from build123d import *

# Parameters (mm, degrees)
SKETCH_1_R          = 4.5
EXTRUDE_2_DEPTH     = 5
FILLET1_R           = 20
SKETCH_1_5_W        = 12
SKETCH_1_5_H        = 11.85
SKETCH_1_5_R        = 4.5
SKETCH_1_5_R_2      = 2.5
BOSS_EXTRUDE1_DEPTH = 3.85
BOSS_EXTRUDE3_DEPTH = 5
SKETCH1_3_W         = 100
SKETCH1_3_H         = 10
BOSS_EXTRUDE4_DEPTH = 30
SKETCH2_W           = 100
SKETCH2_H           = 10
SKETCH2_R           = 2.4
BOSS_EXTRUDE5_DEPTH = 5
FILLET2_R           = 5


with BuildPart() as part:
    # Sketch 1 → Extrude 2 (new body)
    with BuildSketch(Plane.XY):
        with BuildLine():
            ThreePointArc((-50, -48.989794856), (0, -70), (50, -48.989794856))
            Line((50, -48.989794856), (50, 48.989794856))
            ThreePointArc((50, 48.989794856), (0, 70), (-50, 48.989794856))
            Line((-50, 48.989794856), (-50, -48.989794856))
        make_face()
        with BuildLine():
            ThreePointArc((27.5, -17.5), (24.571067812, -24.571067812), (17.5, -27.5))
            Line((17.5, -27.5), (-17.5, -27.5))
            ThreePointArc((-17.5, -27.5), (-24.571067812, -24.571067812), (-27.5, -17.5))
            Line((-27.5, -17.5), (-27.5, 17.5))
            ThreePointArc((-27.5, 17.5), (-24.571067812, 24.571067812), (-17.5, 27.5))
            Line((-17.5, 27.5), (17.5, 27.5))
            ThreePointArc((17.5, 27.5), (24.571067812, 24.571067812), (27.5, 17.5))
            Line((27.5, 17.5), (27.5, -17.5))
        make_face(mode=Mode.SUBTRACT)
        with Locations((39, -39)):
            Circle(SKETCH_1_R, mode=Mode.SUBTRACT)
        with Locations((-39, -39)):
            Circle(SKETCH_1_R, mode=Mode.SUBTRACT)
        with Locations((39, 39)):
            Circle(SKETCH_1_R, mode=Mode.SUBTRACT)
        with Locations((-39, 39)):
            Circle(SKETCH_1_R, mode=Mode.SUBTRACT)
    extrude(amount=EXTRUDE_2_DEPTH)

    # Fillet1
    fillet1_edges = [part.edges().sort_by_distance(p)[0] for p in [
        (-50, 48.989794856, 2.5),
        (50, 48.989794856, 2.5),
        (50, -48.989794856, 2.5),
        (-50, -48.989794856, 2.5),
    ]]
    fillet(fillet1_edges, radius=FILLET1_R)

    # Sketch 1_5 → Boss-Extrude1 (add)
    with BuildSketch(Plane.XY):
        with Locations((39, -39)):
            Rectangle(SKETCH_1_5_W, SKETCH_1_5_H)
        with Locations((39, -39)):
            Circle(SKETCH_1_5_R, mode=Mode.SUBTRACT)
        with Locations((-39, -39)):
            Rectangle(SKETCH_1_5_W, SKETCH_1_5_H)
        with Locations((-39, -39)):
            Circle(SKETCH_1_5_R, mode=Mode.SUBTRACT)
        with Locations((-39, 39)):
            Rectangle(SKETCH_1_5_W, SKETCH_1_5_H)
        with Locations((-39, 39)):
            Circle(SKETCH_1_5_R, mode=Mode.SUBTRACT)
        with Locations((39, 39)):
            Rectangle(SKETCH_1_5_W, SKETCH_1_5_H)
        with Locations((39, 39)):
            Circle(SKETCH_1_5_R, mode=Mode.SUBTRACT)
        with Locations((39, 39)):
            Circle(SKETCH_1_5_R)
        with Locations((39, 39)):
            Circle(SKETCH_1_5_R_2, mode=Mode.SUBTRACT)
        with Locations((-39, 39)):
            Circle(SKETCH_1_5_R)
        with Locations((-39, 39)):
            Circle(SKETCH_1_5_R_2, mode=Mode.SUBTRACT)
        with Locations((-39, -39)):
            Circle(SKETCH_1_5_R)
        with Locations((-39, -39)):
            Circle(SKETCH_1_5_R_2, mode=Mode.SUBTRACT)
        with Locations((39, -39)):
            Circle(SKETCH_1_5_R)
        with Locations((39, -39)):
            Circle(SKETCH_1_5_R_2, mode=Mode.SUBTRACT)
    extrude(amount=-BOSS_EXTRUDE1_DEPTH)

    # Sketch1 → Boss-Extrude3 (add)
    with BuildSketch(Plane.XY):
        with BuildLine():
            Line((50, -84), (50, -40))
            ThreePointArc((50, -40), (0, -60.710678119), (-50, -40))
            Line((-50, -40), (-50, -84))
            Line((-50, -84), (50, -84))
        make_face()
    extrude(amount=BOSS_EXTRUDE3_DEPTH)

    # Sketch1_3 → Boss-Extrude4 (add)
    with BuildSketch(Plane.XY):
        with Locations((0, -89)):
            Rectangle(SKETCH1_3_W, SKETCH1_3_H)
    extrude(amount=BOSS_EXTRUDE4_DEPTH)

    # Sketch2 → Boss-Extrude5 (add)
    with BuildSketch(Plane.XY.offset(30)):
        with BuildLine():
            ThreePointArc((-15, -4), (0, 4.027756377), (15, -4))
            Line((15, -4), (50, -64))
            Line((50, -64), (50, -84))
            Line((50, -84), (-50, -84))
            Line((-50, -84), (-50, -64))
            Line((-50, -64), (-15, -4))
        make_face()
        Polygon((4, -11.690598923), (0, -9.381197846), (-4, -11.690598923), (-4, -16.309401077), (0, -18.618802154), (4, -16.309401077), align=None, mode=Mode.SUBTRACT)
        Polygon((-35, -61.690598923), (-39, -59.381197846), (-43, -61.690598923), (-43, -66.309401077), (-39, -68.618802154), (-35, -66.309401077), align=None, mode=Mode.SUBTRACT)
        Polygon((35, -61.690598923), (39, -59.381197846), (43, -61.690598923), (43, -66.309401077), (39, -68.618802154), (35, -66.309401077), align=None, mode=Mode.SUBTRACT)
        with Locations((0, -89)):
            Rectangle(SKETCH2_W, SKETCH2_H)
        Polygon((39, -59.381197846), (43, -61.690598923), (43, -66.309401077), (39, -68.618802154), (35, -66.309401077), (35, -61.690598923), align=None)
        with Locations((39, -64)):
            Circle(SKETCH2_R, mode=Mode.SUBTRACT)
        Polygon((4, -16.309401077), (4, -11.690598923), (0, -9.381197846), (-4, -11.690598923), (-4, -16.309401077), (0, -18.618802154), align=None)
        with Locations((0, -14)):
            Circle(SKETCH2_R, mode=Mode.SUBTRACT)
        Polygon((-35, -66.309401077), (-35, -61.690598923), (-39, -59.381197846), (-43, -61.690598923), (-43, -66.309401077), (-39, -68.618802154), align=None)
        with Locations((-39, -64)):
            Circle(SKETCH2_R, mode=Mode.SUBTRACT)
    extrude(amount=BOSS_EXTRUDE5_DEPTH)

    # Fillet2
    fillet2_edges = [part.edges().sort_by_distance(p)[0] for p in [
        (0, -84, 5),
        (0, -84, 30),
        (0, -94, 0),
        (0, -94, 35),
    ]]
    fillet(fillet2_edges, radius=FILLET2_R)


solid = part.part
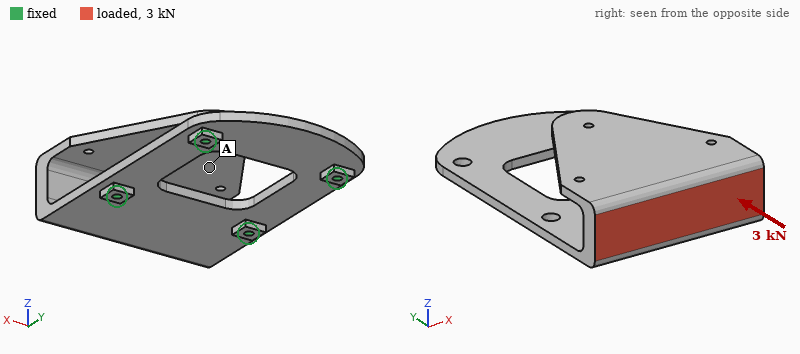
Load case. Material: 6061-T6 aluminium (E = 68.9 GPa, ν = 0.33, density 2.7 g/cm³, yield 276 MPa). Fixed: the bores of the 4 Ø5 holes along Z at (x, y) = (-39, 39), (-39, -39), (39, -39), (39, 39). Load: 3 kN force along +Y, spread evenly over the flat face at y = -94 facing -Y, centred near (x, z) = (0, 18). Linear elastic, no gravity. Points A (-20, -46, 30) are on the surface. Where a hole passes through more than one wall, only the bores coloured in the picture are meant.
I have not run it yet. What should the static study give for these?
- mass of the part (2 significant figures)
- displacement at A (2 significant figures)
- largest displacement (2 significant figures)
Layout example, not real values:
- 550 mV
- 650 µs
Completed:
- 340 g
- 0.99 mm
- 2.3 mm
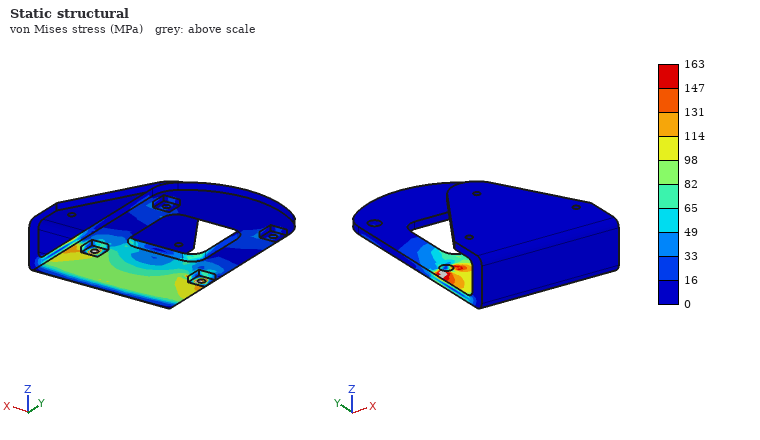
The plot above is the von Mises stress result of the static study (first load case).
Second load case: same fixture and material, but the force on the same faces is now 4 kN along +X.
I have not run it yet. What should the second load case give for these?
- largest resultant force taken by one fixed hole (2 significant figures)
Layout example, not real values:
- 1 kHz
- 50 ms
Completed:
- 3.5 kN
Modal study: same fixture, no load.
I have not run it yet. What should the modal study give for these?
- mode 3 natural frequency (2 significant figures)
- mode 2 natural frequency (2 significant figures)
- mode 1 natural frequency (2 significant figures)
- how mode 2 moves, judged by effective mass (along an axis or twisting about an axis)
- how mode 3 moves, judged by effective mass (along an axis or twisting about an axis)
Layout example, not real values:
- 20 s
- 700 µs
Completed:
- 850 Hz
- 690 Hz
- 370 Hz
- along Z
- along X
